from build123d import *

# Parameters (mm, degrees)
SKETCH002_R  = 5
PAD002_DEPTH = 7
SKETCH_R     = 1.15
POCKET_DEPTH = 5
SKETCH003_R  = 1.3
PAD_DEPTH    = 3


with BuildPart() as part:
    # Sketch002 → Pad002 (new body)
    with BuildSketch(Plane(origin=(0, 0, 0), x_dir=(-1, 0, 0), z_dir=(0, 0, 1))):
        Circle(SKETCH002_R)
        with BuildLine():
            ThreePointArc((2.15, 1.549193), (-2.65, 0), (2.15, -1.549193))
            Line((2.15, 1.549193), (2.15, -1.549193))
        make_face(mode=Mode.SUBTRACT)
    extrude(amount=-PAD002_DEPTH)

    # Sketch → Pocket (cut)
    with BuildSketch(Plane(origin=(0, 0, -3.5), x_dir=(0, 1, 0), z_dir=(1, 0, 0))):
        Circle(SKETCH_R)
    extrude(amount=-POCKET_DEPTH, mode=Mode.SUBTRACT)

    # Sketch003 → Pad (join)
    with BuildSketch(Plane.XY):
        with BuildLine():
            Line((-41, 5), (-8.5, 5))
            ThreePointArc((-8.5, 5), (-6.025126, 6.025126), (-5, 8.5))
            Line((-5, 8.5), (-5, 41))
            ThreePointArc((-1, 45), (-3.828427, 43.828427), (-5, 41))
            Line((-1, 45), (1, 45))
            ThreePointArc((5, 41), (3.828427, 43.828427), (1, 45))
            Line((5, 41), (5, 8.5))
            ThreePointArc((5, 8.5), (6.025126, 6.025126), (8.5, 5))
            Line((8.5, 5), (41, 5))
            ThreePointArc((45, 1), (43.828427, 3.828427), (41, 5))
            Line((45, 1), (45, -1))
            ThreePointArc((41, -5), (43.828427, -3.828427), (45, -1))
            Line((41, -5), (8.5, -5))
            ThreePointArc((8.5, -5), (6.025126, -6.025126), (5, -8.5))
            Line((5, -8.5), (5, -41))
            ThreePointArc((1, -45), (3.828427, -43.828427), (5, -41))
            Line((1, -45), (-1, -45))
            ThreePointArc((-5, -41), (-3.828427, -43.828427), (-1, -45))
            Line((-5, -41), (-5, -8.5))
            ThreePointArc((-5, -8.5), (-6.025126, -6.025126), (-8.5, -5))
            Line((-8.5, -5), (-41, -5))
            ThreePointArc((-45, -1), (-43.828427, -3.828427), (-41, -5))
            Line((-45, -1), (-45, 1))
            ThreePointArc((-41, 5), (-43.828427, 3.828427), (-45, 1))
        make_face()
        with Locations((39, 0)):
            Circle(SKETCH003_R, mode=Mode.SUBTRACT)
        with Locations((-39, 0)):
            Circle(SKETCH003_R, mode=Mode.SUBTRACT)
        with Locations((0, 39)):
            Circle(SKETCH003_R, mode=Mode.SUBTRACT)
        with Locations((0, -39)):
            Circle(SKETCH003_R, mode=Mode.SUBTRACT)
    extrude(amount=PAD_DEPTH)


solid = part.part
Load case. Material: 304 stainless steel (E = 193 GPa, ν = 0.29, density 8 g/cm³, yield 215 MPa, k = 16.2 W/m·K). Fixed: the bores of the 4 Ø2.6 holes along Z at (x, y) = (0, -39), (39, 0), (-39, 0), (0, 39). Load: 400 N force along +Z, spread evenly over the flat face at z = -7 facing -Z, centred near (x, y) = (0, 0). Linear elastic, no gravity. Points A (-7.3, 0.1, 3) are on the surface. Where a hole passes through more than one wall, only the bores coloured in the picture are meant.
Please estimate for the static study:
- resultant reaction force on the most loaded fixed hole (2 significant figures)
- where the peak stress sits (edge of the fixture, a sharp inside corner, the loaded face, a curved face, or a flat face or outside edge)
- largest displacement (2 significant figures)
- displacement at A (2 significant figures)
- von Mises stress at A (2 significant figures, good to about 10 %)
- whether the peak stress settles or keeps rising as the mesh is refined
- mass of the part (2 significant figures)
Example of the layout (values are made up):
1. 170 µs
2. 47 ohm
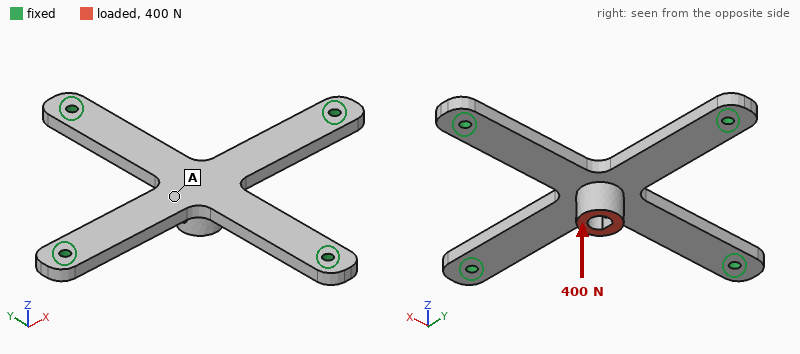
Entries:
1. 100 N
2. edge of the fixture
3. 82 µm
4. 79 µm
5. 74 MPa
6. keeps rising
7. 43 g
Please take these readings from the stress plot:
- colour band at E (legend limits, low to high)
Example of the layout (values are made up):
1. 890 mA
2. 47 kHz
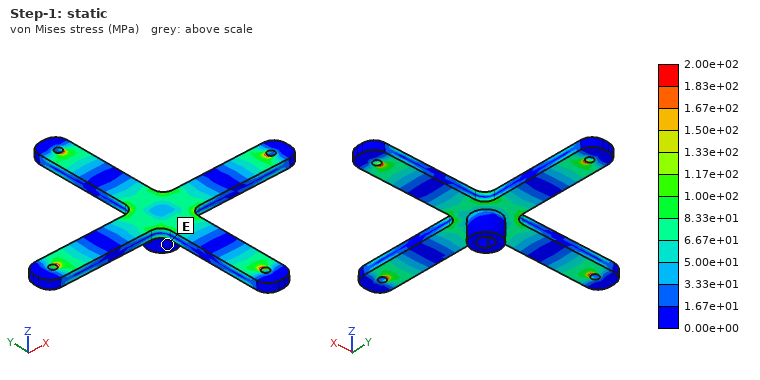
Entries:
1. 0.00e+00 to 1.67e+01 MPa
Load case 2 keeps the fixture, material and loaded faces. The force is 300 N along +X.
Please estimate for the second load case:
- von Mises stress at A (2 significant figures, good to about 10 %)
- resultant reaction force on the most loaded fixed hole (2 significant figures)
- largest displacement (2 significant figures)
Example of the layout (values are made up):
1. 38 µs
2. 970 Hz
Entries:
1. 37 MPa
2. 150 N
3. 17 µm
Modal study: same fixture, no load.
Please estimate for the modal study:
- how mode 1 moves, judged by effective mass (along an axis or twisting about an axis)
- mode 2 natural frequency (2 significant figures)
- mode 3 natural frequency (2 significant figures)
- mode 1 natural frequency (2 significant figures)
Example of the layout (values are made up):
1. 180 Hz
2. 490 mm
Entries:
1. along Z
2. 6900 Hz
3. 6900 Hz
4. 2700 Hz
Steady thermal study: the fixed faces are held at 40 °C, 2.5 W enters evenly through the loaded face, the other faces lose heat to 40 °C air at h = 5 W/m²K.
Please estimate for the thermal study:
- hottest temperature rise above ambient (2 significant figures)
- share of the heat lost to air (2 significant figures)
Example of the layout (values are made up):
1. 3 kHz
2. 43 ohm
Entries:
1. 62 K
2. 18 %
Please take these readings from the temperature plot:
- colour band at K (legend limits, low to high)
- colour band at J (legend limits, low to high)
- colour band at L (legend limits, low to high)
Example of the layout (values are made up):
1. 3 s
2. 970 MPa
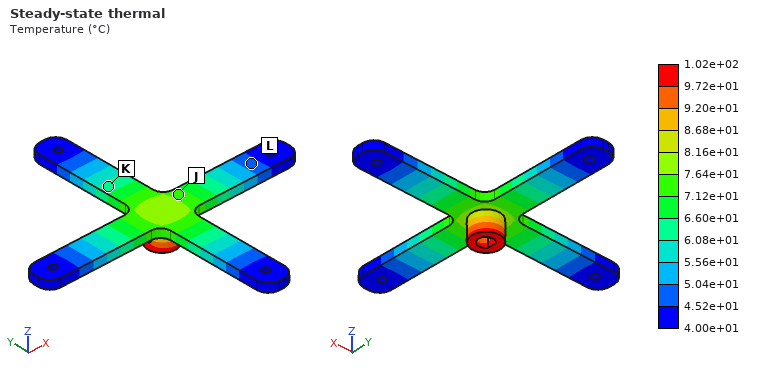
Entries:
1. 6.08e+01 to 6.60e+01 °C
2. 7.12e+01 to 7.64e+01 °C
3. 4.52e+01 to 5.04e+01 °C
